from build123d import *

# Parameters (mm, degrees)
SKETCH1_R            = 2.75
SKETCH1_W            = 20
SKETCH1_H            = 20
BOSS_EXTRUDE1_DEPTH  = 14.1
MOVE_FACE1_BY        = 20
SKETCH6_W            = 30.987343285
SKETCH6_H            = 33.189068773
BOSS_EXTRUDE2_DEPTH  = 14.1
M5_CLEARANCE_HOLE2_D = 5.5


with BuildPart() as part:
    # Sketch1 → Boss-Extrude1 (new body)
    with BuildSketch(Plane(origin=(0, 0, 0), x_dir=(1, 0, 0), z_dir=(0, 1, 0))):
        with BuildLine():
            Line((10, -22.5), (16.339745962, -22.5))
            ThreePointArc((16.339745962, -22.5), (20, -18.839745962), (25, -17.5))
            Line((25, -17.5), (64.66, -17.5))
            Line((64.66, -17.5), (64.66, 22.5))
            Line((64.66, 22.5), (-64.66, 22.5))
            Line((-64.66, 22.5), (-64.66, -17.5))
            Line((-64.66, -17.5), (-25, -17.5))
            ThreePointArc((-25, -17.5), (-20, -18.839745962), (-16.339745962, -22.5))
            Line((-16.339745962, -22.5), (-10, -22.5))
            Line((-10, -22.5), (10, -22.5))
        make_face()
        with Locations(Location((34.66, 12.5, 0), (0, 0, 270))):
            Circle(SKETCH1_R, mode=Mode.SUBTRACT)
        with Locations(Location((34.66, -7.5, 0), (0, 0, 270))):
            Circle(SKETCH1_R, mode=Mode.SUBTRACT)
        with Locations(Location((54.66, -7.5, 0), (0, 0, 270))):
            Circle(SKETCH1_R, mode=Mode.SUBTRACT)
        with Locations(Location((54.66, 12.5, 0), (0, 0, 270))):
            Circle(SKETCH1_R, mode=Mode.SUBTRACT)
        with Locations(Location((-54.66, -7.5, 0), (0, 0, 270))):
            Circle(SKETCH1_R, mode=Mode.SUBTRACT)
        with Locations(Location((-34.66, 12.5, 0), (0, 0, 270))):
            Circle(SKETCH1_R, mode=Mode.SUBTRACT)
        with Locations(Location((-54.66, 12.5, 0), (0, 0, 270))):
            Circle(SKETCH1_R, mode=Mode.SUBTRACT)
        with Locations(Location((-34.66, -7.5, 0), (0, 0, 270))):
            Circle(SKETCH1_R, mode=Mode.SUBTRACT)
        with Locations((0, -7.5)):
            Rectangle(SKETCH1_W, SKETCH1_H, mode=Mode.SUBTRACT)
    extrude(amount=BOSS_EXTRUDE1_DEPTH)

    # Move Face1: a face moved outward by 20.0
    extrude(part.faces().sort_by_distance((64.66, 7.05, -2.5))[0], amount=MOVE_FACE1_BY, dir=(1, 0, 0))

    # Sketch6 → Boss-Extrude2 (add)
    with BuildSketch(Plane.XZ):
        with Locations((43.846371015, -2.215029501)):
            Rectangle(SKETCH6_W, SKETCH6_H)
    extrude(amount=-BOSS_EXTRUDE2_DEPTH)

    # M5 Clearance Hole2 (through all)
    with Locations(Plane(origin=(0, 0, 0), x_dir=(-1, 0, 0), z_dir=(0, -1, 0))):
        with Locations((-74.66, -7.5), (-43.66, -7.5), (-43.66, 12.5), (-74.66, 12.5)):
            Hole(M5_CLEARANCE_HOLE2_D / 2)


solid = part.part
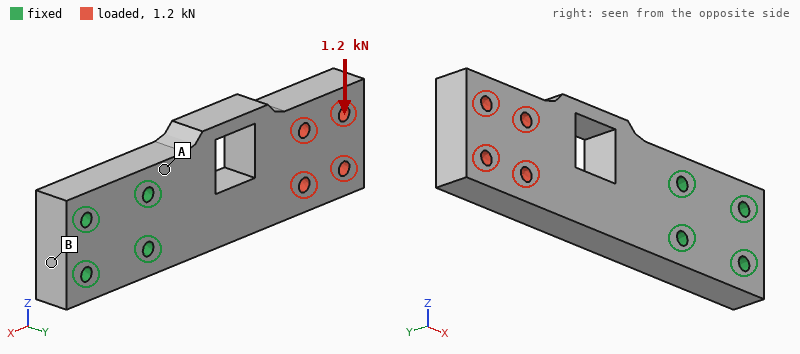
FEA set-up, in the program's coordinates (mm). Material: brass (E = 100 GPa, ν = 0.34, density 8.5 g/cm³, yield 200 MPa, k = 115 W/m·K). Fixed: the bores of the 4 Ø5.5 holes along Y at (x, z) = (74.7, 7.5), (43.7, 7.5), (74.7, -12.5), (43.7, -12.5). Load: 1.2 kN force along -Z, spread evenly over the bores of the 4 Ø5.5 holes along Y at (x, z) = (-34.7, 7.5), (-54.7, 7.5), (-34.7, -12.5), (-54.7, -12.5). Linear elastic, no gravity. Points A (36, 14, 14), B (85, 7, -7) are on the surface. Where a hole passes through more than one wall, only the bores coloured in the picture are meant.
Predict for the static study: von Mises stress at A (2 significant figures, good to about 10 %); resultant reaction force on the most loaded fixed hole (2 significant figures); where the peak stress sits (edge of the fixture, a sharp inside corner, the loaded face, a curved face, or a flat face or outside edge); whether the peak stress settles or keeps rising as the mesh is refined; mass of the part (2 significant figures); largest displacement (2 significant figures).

18 MPa
3.8 kN
edge of the fixture
keeps rising
670 g
73 µm
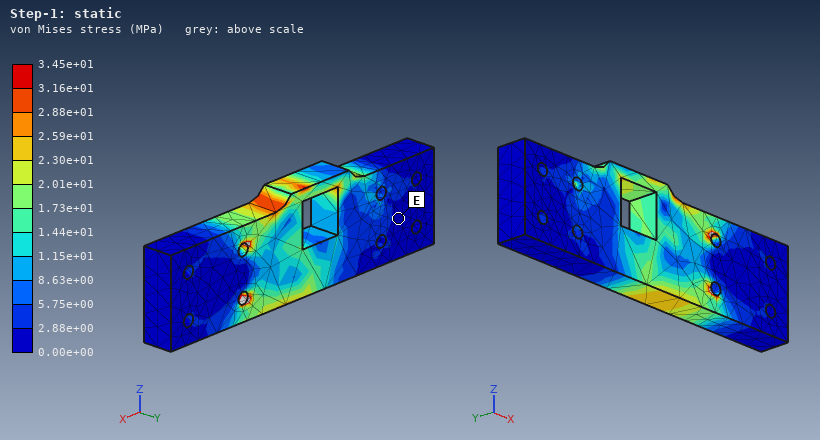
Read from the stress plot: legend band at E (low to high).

0.00e+00 to 2.88e+00 MPa
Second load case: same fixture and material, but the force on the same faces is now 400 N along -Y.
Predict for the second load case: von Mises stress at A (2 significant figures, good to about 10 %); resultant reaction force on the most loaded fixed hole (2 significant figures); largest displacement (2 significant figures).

20 MPa
310 N
0.16 mm
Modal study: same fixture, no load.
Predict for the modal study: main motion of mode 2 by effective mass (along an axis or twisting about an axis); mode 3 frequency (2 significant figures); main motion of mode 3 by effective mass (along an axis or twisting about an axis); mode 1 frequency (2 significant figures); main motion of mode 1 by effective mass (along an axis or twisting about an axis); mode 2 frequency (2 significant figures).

along Z
2700 Hz
twisting about X
630 Hz
along Y
1500 Hz
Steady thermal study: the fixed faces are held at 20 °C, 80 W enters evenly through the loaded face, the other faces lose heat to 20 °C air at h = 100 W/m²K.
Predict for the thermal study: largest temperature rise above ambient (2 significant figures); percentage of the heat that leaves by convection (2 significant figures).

69 K
60 %
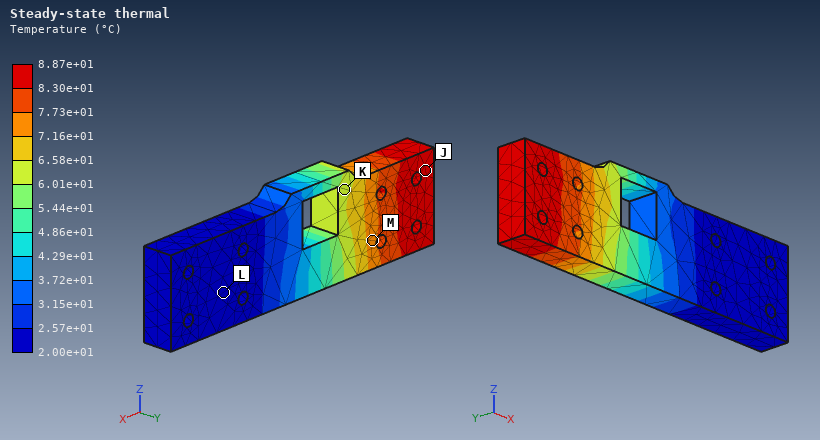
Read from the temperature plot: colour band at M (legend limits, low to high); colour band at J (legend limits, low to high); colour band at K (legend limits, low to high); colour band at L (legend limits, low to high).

7.16e+01 to 7.73e+01 °C
8.30e+01 to 8.87e+01 °C
6.01e+01 to 6.58e+01 °C
2.00e+01 to 2.57e+01 °C
